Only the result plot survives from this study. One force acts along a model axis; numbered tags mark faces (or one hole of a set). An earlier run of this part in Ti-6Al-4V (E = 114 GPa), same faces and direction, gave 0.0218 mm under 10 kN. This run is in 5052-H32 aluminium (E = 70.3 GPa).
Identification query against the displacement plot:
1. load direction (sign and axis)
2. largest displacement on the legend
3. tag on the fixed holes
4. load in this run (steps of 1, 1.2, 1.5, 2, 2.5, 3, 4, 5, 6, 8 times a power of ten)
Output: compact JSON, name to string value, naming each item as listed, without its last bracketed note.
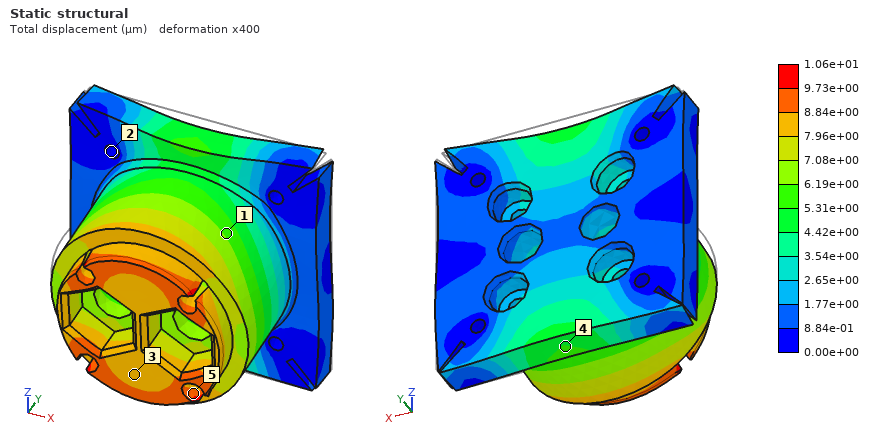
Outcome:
{"load direction": "-Z", "largest displacement on the legend": "1.06e+01 µm", "tag on the fixed holes": "2", "load in this run": "3 kN"}
